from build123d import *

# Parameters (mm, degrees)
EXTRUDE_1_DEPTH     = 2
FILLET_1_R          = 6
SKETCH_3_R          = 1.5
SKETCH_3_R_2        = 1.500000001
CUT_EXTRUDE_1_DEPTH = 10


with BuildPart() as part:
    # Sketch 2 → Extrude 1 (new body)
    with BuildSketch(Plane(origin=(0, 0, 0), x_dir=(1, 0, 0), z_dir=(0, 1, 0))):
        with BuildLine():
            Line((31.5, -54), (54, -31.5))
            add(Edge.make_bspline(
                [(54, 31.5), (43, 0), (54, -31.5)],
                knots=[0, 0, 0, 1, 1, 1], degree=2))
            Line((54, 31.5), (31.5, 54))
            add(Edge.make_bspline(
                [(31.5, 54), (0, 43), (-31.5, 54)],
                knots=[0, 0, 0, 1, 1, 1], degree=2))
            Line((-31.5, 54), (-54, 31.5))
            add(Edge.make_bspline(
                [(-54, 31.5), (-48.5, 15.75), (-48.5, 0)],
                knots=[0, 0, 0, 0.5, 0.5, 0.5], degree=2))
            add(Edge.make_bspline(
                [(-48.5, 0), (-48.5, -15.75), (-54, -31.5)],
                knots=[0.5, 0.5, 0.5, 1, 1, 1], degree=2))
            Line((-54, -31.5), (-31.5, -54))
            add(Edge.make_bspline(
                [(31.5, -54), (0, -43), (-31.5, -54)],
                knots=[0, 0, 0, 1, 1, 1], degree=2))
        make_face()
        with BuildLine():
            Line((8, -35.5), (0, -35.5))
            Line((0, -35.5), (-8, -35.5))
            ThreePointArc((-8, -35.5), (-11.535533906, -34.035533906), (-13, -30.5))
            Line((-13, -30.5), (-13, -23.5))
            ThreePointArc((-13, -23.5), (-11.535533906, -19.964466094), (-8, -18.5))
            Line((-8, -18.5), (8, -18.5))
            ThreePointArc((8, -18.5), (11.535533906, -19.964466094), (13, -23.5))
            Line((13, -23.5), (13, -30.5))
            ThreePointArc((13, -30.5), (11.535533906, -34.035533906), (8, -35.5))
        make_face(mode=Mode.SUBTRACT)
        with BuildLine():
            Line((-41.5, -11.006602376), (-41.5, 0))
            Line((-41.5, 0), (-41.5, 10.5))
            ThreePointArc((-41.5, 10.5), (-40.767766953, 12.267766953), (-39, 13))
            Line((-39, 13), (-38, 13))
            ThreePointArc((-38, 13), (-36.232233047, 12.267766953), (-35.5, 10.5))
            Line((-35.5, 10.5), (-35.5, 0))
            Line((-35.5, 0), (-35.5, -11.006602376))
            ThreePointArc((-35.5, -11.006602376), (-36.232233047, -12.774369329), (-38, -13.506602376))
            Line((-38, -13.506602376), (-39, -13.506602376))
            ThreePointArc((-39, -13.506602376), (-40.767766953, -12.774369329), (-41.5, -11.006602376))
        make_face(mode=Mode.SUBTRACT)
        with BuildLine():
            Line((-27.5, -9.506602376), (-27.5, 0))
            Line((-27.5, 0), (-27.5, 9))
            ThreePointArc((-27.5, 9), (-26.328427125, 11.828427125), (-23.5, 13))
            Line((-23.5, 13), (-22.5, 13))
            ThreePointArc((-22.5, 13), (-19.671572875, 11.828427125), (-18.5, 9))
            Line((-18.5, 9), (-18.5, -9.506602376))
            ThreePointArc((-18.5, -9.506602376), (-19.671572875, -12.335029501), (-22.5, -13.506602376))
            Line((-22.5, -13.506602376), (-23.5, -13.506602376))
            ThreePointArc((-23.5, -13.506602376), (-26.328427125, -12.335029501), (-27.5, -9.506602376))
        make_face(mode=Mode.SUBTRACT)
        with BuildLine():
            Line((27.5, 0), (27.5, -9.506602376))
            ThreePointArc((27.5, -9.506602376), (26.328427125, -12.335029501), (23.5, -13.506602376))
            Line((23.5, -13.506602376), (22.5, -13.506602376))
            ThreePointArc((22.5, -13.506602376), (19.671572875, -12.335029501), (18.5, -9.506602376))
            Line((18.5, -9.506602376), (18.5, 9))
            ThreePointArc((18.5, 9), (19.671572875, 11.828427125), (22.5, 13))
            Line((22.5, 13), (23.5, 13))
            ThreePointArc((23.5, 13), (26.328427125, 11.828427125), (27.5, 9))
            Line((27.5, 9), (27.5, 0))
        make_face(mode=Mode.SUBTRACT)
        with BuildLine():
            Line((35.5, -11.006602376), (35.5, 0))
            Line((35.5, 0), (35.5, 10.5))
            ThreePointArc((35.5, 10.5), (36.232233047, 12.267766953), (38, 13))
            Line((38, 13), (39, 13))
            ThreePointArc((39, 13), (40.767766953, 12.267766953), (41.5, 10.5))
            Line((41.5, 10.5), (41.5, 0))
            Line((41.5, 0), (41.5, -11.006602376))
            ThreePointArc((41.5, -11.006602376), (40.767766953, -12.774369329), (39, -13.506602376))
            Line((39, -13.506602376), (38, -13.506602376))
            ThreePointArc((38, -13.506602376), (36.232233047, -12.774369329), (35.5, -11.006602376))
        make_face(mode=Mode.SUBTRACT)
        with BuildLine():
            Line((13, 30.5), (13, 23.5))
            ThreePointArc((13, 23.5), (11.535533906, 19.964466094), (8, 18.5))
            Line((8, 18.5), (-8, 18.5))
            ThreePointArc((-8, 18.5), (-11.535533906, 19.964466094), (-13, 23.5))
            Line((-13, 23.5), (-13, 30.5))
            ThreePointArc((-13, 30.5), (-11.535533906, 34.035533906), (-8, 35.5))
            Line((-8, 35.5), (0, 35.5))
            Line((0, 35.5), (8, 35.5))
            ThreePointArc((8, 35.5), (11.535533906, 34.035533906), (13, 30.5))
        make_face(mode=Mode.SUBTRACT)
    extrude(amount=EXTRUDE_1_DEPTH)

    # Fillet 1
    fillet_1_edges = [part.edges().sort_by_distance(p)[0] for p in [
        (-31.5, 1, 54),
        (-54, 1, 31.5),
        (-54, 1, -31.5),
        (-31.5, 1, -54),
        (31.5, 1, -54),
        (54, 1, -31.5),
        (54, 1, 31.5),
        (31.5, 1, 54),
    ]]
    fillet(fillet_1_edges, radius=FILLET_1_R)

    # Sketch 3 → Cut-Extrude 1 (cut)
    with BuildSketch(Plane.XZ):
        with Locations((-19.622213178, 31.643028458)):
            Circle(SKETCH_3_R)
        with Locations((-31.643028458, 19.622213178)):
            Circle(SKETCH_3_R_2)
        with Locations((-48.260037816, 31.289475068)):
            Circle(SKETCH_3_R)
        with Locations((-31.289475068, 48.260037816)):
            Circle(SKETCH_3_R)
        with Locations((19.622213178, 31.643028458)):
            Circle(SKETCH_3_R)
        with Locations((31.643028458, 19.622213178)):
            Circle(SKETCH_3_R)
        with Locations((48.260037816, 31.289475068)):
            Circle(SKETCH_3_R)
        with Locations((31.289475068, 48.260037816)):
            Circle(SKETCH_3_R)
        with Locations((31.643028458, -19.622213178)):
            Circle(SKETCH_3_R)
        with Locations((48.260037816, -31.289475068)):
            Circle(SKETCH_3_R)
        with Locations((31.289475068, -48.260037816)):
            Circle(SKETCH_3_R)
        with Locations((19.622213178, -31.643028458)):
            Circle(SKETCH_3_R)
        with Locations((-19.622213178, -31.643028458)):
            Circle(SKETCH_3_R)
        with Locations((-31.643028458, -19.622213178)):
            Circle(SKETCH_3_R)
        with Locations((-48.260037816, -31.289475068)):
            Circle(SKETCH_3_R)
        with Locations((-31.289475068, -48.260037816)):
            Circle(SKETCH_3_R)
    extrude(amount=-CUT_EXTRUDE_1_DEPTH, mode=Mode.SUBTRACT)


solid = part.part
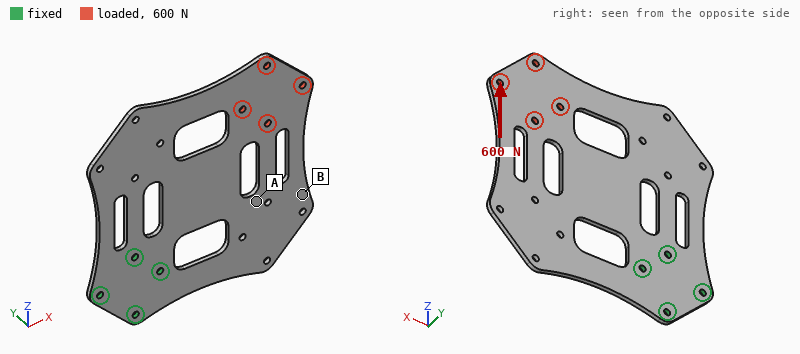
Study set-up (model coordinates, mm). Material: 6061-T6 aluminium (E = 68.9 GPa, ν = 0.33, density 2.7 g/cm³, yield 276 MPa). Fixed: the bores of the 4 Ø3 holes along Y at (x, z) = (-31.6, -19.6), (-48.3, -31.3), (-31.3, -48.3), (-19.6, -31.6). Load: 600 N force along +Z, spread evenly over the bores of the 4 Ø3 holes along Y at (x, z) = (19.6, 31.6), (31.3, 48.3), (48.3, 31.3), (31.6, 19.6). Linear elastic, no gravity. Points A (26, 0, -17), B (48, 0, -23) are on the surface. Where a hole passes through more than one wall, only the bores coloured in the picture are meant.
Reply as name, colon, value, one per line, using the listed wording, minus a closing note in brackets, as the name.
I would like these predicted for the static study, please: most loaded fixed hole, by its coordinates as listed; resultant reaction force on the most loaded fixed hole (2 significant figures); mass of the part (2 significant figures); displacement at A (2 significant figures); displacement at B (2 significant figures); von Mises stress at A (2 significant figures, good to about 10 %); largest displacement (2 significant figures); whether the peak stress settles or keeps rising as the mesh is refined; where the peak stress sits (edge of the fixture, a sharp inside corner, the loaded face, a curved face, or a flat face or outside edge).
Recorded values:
most loaded fixed hole, by its coordinates as listed: (-19.6, -31.6)
resultant reaction force on the most loaded fixed hole: 1.0 kN
mass of the part: 43 g
displacement at A: 0.091 mm
displacement at B: 0.12 mm
von Mises stress at A: 18 MPa
largest displacement: 0.17 mm
whether the peak stress settles or keeps rising as the mesh is refined: keeps rising
where the peak stress sits: edge of the fixture
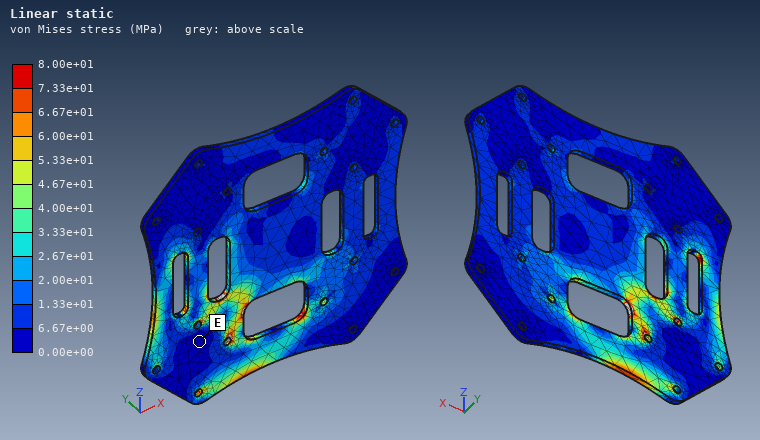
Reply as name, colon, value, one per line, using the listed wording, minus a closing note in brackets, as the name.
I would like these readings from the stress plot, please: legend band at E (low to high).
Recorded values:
legend band at E: 0.00e+00 to 6.67e+00 MPa
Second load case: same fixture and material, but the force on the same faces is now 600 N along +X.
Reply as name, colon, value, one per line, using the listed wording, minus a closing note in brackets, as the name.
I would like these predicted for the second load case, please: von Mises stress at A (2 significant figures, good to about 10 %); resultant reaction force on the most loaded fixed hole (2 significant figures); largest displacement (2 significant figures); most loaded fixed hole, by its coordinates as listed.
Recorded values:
von Mises stress at A: 10 MPa
resultant reaction force on the most loaded fixed hole: 960 N
largest displacement: 0.17 mm
most loaded fixed hole, by its coordinates as listed: (-31.6, -19.6)
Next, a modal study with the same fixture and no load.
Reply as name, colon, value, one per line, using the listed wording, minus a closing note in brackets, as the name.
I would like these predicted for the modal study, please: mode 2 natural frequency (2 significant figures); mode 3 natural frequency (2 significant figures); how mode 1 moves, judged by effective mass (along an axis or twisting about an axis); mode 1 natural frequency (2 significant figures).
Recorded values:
mode 2 natural frequency: 310 Hz
mode 3 natural frequency: 590 Hz
how mode 1 moves, judged by effective mass: along Y
mode 1 natural frequency: 160 Hz
